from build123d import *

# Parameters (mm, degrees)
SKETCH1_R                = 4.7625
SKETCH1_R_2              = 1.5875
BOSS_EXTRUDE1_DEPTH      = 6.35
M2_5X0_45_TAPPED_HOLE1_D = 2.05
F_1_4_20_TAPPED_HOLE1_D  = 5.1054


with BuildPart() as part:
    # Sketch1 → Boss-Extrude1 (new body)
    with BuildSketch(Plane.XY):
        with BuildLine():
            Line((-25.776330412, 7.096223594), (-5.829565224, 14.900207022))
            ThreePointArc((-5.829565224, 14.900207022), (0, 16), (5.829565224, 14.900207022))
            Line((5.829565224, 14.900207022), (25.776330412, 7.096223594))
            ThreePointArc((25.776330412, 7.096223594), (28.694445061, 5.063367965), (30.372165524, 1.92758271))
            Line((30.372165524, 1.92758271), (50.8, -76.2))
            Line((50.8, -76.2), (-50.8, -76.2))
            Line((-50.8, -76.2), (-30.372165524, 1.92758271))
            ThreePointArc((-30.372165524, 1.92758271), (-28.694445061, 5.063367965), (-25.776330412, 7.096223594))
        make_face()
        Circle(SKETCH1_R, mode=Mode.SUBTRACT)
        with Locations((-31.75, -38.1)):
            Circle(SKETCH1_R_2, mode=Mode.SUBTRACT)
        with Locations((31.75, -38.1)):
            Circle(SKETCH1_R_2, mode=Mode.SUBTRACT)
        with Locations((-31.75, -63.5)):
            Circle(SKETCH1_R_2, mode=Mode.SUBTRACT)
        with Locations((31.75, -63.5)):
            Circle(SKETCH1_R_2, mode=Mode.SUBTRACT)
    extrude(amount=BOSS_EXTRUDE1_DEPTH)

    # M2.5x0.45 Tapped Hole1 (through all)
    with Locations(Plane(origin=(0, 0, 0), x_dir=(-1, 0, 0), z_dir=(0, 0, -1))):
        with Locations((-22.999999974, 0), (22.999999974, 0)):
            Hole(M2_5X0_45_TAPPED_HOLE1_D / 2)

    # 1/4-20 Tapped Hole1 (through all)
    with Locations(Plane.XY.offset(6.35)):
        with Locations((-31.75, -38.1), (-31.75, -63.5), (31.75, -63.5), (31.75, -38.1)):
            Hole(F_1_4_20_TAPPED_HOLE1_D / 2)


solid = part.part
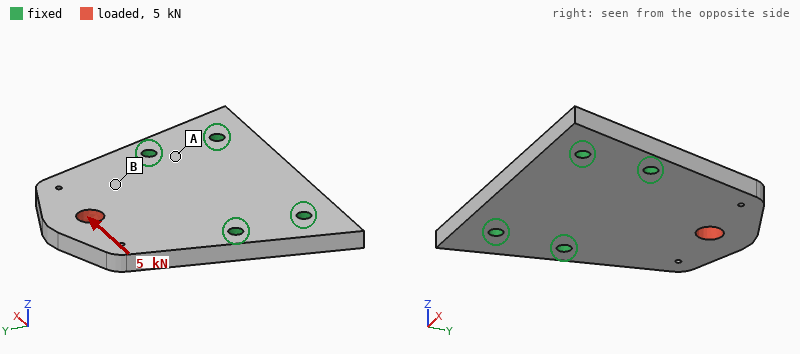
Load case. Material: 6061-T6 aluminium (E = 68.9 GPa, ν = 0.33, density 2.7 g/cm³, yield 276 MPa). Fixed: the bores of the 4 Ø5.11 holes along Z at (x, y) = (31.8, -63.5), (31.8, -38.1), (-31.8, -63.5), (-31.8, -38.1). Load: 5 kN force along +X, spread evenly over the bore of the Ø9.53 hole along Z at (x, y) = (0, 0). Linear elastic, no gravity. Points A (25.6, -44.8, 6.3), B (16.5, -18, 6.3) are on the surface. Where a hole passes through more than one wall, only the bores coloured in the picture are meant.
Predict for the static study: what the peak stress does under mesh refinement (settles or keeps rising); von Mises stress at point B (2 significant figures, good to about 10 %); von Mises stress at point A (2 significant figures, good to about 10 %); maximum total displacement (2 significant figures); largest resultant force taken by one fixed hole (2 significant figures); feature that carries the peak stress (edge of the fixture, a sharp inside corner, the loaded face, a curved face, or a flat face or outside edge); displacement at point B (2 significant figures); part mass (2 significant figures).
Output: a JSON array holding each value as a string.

["keeps rising", "22 MPa", "6.6 MPa", "32 µm", "3.4 kN", "edge of the fixture", "12 µm", "120 g"]
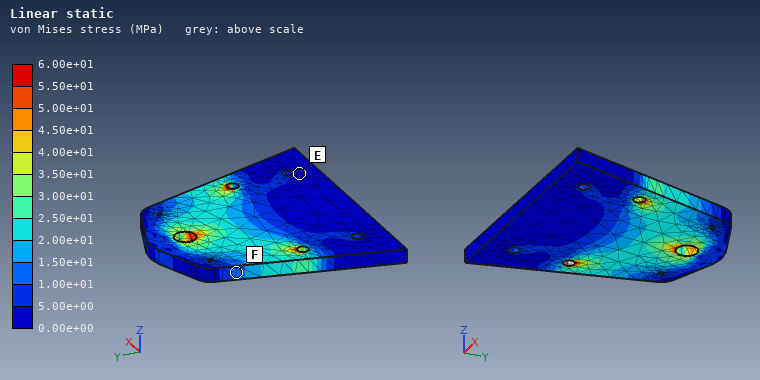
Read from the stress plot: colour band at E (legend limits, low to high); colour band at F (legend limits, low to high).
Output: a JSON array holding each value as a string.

["0.00e+00 to 5.00e+00 MPa", "1.00e+01 to 1.50e+01 MPa"]
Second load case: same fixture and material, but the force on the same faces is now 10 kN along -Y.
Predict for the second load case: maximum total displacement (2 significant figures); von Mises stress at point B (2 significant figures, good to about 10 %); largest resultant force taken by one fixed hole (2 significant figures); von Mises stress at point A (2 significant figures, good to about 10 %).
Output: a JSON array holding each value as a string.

["34 µm", "30 MPa", "3.7 kN", "22 MPa"]
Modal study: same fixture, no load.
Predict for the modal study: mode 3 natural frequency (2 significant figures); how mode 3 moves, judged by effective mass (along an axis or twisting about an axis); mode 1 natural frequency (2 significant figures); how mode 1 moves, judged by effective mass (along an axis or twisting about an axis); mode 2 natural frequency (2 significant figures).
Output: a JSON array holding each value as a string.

["7500 Hz", "along Z", "2000 Hz", "along Z", "5100 Hz"]
